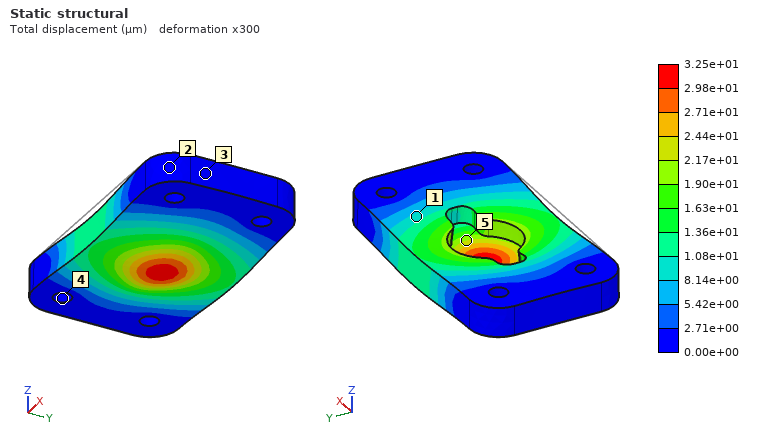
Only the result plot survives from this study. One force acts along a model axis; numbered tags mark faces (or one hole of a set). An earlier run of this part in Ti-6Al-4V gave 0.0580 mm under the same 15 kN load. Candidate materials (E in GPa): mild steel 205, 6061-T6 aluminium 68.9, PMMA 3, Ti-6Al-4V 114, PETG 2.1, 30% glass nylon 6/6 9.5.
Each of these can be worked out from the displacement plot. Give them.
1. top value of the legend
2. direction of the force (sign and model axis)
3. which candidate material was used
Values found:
3.25e+01 µm
-Z
mild steel
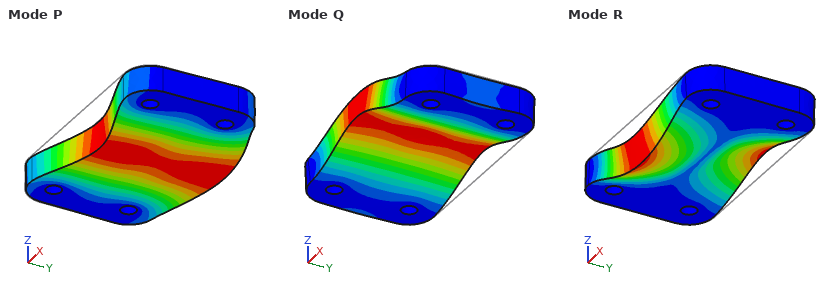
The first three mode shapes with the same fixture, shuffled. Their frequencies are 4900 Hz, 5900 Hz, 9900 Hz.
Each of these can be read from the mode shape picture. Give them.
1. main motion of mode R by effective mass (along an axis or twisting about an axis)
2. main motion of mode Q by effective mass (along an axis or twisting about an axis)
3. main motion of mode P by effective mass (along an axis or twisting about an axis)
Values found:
twisting about X
along Z
along Y
